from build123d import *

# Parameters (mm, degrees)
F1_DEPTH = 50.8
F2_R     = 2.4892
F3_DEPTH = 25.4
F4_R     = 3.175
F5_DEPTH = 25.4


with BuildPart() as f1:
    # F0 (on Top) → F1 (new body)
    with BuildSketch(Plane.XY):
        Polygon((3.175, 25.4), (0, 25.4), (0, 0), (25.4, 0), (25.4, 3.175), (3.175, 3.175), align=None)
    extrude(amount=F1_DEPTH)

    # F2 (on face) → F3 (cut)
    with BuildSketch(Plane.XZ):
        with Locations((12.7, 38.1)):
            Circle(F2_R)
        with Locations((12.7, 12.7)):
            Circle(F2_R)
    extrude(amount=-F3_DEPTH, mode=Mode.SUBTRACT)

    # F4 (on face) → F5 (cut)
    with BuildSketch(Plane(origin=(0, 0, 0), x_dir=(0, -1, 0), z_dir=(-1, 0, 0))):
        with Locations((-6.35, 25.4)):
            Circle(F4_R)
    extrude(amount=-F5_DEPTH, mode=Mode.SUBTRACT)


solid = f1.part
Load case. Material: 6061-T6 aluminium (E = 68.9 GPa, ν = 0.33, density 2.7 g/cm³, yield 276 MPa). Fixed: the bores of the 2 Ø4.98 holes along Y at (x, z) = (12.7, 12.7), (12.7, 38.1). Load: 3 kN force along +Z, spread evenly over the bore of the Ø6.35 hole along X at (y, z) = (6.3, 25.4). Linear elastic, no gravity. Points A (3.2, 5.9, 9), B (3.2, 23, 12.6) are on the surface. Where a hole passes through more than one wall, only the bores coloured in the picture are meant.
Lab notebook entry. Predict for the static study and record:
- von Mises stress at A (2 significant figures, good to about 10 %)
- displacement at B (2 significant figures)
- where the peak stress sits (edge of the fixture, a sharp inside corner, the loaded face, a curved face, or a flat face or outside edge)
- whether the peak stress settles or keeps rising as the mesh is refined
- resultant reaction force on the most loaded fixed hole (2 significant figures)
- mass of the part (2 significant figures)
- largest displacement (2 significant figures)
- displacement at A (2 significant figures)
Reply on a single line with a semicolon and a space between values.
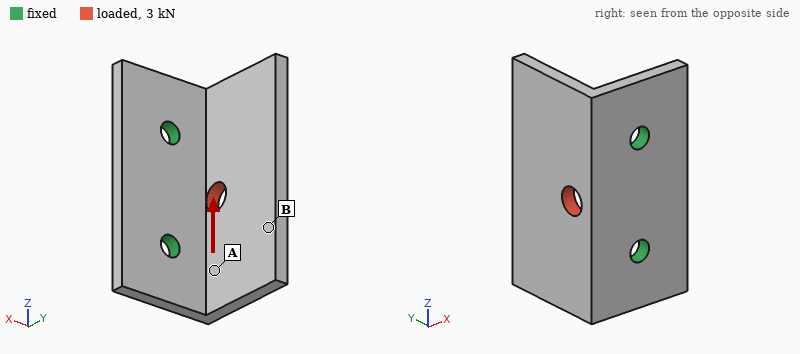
42 MPa; 72 µm; edge of the fixture; keeps rising; 1.9 kN; 20 g; 99 µm; 37 µm
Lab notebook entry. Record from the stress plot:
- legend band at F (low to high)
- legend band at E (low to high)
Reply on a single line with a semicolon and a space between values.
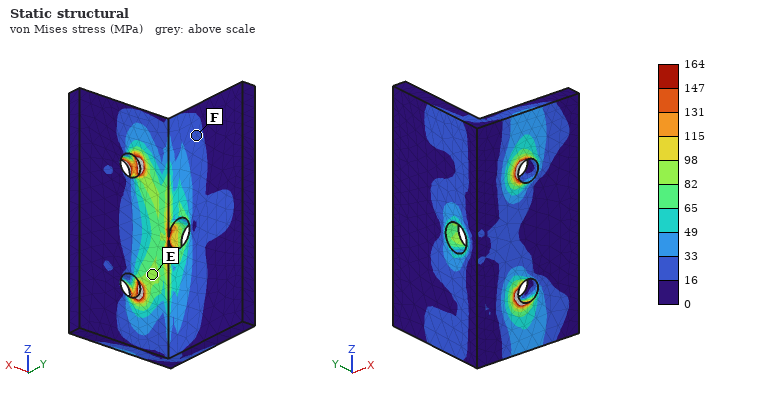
16 to 33 MPa; 82 to 98 MPa
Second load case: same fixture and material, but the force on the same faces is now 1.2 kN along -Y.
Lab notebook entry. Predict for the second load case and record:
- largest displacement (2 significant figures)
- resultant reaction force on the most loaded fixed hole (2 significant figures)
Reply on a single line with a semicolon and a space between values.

0.19 mm; 600 N
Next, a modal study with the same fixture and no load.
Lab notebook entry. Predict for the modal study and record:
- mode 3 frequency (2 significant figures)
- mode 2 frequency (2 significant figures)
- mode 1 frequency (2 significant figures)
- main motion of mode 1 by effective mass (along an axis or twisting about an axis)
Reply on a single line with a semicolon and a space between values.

7500 Hz; 4600 Hz; 2700 Hz; along X
